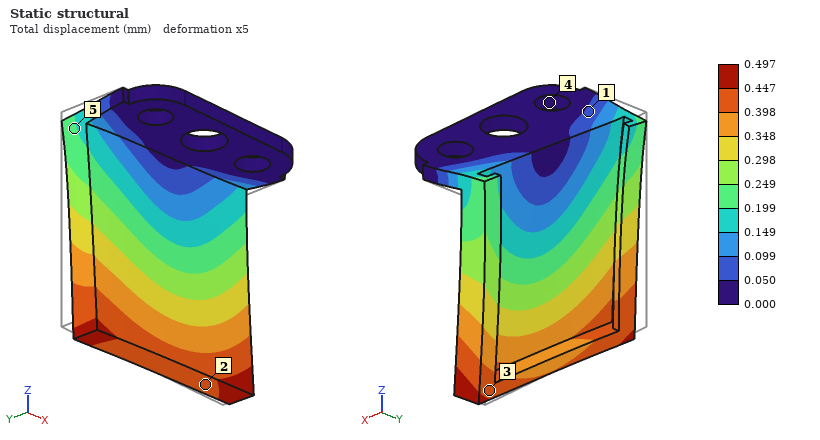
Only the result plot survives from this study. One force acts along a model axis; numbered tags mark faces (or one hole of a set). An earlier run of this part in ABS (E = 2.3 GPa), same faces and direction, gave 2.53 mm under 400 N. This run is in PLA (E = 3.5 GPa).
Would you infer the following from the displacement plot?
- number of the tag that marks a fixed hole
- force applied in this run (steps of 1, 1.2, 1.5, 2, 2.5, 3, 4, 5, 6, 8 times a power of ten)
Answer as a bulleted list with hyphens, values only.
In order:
- 4
- 120 N
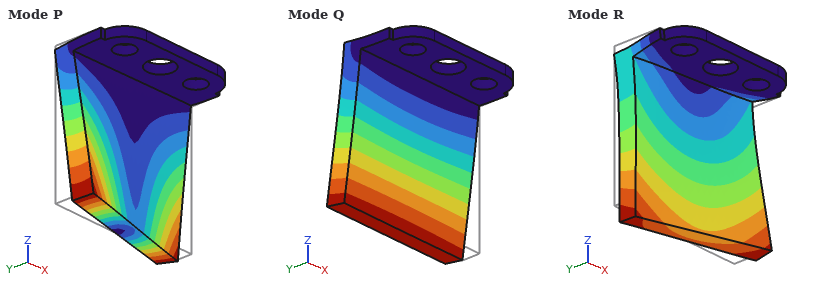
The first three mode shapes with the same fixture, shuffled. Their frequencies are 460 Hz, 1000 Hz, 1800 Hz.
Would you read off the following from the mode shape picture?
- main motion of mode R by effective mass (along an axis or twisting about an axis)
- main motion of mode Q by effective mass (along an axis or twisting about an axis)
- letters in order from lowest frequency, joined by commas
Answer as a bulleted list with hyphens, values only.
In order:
- along X
- along Y
- Q, P, R
